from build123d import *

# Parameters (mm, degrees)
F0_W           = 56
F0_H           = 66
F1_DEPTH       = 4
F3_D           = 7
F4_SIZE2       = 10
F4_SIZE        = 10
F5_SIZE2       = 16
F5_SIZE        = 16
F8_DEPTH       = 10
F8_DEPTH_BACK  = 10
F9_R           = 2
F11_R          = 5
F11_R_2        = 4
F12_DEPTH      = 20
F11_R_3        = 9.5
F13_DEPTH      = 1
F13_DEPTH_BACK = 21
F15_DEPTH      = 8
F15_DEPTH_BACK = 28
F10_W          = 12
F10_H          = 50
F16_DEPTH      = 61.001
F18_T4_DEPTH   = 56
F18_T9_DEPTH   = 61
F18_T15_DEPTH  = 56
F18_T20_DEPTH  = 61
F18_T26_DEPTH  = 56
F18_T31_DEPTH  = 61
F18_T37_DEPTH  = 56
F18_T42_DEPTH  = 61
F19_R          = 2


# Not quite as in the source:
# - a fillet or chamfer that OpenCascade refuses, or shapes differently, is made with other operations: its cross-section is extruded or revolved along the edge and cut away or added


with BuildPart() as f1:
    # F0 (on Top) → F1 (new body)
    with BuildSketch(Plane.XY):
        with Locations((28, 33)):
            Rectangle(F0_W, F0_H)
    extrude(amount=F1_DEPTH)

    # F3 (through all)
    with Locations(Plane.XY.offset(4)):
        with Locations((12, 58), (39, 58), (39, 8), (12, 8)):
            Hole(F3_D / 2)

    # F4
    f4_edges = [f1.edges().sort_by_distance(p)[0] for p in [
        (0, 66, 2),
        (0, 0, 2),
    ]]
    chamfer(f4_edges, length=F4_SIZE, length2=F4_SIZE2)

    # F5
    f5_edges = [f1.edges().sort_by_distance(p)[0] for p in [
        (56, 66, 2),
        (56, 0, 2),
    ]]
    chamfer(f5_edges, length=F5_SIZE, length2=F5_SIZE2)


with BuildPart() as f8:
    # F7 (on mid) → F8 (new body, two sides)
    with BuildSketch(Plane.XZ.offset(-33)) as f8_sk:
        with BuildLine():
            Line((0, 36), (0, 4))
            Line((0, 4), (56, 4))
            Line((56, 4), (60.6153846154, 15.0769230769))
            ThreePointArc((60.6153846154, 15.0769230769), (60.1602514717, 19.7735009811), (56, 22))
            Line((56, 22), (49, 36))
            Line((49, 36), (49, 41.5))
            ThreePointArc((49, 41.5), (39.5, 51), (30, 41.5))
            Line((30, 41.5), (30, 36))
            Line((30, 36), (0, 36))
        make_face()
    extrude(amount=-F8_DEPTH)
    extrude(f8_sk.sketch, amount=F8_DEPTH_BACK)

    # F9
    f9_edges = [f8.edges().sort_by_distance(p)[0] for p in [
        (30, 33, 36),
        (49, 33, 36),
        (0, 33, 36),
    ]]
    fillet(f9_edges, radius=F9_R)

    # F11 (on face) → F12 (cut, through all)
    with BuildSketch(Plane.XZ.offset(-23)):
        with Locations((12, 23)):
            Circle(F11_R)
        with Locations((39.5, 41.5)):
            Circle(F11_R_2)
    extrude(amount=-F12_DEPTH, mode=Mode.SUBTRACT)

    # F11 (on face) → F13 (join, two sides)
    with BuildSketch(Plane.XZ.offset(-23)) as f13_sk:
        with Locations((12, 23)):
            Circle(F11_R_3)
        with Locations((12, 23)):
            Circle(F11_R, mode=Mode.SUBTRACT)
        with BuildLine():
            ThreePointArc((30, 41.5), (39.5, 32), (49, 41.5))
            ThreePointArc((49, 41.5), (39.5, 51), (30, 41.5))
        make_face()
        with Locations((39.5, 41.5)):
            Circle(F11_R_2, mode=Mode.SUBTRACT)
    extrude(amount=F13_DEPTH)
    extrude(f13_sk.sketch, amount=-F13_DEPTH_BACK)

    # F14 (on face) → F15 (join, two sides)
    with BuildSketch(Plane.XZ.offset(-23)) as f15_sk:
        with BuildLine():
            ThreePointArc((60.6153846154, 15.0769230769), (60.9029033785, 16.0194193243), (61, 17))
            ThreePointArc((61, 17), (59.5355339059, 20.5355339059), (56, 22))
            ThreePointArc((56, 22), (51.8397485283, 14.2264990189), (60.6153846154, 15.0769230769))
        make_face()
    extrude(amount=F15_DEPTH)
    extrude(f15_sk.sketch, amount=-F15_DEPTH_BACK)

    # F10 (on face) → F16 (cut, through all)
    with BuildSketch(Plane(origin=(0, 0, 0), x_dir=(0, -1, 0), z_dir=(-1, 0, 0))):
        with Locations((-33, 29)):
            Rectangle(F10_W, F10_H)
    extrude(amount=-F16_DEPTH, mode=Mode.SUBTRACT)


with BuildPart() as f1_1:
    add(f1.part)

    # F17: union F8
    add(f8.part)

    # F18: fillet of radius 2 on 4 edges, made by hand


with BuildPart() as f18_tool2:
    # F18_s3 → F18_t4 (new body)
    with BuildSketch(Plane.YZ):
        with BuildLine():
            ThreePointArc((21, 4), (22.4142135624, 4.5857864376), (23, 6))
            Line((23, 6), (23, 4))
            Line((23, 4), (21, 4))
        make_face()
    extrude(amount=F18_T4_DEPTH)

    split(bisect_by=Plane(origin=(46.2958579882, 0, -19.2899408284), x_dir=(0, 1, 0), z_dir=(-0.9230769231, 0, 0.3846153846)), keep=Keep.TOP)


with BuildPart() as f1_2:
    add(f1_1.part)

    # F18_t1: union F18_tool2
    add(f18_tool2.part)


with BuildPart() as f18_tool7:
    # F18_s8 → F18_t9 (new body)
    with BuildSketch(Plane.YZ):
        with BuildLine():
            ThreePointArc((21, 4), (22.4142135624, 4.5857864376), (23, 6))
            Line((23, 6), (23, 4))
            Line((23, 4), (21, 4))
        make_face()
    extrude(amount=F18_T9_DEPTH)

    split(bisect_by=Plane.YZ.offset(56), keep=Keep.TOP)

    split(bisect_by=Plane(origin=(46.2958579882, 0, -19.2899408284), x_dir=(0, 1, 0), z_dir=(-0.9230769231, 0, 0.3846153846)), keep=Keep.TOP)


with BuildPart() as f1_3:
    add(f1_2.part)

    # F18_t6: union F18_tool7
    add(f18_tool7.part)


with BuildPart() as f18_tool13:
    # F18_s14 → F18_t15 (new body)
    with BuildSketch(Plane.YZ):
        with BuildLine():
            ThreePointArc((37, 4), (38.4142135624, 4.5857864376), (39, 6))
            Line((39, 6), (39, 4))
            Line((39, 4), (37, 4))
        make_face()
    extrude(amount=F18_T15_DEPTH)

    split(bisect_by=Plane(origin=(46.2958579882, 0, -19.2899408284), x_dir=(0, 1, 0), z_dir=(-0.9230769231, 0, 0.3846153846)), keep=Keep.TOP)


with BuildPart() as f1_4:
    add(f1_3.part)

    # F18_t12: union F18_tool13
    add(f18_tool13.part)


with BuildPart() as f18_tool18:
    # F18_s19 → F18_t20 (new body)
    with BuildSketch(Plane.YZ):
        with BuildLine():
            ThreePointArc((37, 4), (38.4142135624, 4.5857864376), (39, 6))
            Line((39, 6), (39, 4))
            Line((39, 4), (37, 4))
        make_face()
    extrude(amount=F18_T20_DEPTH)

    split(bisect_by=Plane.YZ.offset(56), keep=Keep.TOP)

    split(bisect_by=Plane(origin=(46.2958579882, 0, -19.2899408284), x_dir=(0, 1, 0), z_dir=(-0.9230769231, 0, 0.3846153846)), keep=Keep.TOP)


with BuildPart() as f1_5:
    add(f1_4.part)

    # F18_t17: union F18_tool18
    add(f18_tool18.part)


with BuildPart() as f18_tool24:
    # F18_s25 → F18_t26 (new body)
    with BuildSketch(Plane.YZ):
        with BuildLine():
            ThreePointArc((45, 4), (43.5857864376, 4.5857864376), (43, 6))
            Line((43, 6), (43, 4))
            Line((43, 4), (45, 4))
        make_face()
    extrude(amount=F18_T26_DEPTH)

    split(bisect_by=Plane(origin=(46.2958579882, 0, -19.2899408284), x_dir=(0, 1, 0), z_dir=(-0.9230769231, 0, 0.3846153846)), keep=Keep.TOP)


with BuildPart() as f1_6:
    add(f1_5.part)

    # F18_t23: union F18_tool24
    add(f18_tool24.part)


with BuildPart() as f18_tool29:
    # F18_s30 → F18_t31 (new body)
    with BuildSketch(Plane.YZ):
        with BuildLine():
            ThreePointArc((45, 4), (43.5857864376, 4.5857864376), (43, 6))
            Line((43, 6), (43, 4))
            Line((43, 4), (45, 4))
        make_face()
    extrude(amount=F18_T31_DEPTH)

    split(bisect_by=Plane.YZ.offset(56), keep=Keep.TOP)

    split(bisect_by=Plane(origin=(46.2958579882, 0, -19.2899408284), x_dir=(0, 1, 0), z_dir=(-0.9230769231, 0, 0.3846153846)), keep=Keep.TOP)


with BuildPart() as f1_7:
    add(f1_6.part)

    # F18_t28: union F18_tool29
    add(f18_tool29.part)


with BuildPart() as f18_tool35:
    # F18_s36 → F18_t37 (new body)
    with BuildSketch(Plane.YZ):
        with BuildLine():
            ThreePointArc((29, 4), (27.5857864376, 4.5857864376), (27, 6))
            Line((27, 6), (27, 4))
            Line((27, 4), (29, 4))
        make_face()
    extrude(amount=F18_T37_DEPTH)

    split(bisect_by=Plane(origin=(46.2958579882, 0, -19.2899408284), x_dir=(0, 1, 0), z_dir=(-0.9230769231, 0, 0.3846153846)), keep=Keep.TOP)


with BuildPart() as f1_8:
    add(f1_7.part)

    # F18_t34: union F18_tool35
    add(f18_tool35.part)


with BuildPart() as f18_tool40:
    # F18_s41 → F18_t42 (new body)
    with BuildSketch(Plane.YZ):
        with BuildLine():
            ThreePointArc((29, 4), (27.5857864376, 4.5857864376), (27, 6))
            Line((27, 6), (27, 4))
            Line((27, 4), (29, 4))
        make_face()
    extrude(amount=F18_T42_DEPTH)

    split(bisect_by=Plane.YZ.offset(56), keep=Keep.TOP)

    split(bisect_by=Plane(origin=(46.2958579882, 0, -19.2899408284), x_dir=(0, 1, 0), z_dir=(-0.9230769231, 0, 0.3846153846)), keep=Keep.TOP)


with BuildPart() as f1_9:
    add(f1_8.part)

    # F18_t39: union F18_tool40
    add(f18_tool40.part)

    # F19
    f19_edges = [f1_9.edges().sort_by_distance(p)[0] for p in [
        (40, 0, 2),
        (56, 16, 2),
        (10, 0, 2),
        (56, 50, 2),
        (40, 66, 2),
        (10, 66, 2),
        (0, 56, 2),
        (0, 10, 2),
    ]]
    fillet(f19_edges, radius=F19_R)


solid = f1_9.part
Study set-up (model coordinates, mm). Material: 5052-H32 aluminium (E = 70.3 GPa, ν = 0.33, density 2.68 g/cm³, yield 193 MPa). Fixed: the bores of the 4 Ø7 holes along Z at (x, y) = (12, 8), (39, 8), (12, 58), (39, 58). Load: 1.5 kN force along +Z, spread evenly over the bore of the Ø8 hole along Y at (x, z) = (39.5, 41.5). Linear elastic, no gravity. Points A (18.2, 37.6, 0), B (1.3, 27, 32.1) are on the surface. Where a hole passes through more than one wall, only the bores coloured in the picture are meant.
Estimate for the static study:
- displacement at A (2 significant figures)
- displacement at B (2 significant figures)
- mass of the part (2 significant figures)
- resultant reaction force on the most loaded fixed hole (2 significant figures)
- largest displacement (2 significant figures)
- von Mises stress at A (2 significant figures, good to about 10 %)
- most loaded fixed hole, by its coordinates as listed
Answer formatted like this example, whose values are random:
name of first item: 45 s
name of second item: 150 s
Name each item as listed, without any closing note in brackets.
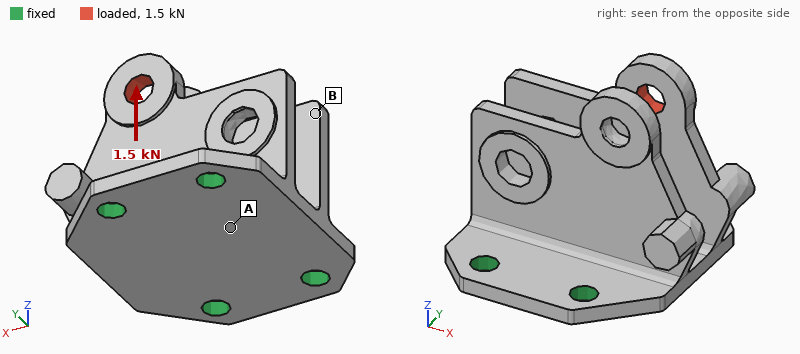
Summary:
displacement at A: 0.019 mm
displacement at B: 0.037 mm
mass of the part: 81 g
resultant reaction force on the most loaded fixed hole: 1.0 kN
largest displacement: 0.10 mm
von Mises stress at A: 20 MPa
most loaded fixed hole, by its coordinates as listed: (39, 58)
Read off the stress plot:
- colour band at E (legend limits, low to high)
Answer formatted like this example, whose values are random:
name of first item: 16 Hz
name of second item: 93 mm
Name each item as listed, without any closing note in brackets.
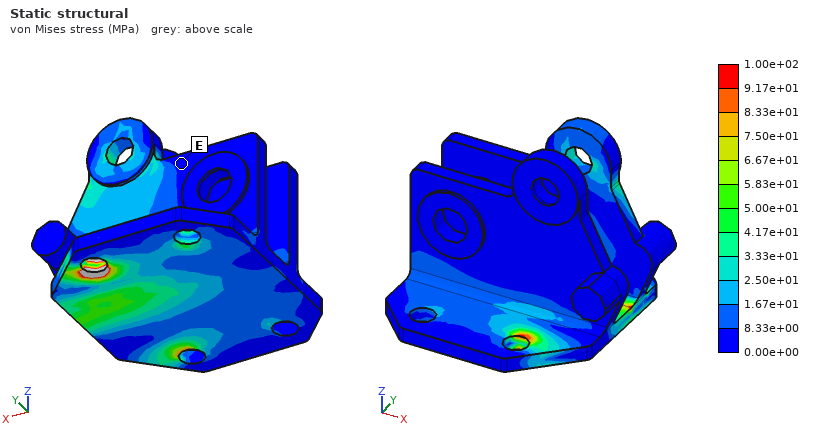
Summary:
colour band at E: 0.00e+00 to 8.33e+00 MPa
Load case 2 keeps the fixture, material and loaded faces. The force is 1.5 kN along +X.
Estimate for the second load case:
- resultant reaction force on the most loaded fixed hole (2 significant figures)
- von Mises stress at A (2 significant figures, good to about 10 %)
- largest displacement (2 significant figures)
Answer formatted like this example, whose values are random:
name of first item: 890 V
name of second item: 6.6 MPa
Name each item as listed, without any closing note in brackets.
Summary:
resultant reaction force on the most loaded fixed hole: 1.4 kN
von Mises stress at A: 38 MPa
largest displacement: 0.24 mm
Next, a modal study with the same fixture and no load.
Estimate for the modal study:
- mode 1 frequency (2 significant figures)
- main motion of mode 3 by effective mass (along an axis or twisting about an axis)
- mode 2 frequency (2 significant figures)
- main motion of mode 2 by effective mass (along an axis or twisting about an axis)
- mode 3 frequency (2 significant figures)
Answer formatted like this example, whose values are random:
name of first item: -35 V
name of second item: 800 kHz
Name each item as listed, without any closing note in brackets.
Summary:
mode 1 frequency: 1900 Hz
main motion of mode 3 by effective mass: along X
mode 2 frequency: 2200 Hz
main motion of mode 2 by effective mass: along Y
mode 3 frequency: 3200 Hz
